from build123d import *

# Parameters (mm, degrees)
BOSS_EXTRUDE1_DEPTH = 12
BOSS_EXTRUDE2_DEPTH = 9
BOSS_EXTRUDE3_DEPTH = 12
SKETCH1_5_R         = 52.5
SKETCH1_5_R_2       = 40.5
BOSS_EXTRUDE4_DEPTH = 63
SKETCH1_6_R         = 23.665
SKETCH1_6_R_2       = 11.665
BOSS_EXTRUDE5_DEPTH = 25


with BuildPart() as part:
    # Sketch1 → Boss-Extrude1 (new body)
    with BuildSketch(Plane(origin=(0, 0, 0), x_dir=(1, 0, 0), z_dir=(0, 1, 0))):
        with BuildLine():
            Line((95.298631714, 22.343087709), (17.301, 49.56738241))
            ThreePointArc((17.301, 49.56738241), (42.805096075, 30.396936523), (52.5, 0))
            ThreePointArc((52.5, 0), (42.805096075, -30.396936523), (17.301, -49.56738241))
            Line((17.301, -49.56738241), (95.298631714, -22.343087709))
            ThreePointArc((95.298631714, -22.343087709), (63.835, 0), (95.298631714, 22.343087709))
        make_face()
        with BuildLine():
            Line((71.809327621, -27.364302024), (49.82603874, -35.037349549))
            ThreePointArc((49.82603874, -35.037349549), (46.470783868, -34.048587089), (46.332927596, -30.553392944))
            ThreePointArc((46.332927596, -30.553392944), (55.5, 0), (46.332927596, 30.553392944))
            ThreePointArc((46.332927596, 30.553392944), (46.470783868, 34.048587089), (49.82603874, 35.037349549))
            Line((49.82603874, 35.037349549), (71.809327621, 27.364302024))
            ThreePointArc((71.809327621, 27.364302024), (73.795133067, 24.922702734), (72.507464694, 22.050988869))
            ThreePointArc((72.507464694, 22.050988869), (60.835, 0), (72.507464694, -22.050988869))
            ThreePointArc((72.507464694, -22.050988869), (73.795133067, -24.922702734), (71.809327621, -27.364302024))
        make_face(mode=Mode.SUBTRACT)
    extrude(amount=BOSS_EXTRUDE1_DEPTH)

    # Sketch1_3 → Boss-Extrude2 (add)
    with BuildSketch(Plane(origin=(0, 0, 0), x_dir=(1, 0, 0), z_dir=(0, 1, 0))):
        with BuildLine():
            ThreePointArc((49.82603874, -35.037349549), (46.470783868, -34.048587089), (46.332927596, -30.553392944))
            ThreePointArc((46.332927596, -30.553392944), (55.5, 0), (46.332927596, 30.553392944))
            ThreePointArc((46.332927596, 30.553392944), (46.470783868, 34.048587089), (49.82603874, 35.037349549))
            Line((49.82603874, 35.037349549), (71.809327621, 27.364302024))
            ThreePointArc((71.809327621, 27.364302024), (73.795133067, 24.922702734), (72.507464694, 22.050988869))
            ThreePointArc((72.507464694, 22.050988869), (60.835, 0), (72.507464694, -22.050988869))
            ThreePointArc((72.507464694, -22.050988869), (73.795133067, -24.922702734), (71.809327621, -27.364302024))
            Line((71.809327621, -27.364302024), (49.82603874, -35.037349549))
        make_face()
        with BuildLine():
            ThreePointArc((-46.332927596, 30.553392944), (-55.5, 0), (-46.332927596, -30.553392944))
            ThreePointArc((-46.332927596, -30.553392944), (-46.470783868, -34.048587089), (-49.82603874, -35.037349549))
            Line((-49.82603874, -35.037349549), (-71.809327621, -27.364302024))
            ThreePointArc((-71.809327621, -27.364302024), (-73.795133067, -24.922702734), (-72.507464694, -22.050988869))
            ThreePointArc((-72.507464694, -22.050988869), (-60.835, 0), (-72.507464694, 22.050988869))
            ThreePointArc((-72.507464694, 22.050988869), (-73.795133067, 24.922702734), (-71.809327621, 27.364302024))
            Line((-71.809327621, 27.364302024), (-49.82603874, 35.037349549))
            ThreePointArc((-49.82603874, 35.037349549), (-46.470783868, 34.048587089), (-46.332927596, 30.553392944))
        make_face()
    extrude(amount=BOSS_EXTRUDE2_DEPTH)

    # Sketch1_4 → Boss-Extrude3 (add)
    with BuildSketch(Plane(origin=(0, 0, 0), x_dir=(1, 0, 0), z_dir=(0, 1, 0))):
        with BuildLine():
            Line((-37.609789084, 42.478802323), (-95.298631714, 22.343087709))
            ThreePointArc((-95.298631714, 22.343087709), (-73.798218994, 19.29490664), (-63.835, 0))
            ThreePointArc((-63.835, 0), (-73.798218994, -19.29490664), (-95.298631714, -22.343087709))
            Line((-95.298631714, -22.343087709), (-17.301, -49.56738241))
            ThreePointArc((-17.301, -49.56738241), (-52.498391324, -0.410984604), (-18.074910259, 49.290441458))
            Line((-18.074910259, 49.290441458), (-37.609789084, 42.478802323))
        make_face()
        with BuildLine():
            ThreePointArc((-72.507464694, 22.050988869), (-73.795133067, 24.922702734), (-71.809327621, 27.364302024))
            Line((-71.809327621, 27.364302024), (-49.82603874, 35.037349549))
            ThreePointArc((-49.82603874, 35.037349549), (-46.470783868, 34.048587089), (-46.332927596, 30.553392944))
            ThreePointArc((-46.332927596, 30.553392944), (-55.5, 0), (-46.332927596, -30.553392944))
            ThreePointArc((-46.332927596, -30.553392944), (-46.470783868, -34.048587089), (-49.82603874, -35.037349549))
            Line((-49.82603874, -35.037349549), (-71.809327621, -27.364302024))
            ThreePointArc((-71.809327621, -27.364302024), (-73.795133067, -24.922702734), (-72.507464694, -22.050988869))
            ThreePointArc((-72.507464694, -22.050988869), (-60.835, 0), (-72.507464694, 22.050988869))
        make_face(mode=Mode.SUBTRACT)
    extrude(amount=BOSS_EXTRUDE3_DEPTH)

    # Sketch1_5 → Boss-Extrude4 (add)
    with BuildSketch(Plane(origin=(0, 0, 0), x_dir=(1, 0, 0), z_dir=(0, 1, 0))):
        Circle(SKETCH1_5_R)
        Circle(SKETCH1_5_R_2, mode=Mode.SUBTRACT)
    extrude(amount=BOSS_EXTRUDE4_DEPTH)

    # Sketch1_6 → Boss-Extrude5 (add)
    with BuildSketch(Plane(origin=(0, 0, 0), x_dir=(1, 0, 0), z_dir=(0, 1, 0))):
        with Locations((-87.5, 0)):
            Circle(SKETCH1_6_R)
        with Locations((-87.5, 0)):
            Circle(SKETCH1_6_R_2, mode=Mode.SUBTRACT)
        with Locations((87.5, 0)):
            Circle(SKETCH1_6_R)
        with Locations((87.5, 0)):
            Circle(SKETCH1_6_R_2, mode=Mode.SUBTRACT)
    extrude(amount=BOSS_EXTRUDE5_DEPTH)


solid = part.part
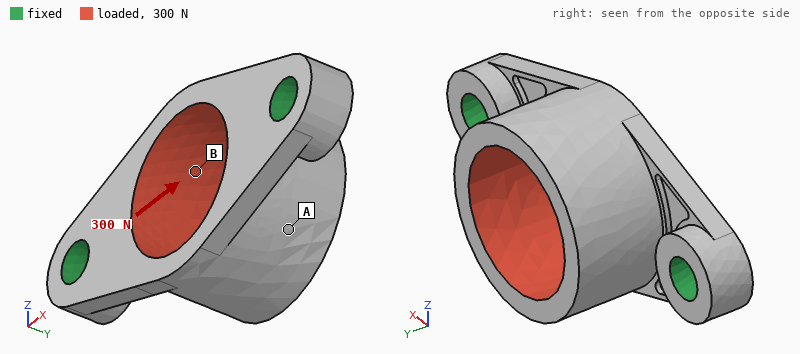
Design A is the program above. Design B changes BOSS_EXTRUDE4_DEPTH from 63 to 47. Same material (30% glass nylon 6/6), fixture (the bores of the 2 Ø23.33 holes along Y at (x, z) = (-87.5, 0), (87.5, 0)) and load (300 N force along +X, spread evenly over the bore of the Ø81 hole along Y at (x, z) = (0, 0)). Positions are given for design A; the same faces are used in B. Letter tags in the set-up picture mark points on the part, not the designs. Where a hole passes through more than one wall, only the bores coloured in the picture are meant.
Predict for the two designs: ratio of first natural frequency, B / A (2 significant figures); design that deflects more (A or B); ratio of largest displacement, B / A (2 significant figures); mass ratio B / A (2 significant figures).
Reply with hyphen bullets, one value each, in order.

- 1.3
- A
- 0.69
- 0.83
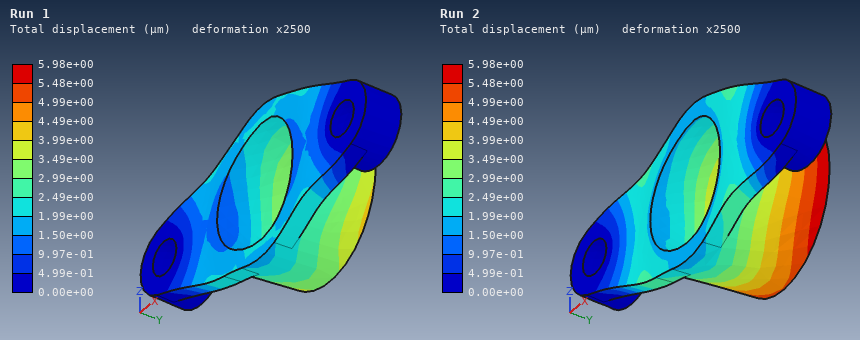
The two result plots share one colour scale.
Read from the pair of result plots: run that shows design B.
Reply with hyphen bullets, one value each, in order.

- Run 1
